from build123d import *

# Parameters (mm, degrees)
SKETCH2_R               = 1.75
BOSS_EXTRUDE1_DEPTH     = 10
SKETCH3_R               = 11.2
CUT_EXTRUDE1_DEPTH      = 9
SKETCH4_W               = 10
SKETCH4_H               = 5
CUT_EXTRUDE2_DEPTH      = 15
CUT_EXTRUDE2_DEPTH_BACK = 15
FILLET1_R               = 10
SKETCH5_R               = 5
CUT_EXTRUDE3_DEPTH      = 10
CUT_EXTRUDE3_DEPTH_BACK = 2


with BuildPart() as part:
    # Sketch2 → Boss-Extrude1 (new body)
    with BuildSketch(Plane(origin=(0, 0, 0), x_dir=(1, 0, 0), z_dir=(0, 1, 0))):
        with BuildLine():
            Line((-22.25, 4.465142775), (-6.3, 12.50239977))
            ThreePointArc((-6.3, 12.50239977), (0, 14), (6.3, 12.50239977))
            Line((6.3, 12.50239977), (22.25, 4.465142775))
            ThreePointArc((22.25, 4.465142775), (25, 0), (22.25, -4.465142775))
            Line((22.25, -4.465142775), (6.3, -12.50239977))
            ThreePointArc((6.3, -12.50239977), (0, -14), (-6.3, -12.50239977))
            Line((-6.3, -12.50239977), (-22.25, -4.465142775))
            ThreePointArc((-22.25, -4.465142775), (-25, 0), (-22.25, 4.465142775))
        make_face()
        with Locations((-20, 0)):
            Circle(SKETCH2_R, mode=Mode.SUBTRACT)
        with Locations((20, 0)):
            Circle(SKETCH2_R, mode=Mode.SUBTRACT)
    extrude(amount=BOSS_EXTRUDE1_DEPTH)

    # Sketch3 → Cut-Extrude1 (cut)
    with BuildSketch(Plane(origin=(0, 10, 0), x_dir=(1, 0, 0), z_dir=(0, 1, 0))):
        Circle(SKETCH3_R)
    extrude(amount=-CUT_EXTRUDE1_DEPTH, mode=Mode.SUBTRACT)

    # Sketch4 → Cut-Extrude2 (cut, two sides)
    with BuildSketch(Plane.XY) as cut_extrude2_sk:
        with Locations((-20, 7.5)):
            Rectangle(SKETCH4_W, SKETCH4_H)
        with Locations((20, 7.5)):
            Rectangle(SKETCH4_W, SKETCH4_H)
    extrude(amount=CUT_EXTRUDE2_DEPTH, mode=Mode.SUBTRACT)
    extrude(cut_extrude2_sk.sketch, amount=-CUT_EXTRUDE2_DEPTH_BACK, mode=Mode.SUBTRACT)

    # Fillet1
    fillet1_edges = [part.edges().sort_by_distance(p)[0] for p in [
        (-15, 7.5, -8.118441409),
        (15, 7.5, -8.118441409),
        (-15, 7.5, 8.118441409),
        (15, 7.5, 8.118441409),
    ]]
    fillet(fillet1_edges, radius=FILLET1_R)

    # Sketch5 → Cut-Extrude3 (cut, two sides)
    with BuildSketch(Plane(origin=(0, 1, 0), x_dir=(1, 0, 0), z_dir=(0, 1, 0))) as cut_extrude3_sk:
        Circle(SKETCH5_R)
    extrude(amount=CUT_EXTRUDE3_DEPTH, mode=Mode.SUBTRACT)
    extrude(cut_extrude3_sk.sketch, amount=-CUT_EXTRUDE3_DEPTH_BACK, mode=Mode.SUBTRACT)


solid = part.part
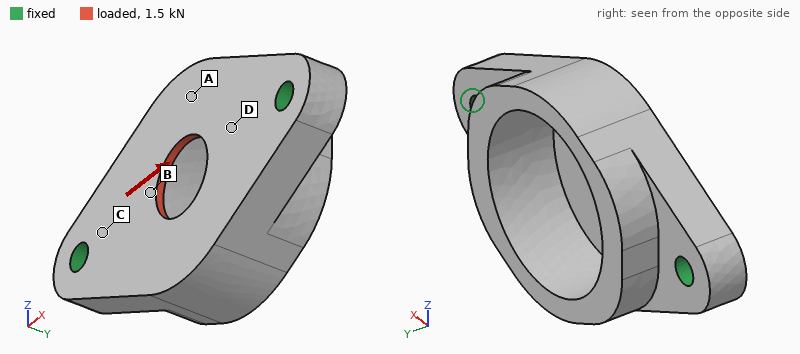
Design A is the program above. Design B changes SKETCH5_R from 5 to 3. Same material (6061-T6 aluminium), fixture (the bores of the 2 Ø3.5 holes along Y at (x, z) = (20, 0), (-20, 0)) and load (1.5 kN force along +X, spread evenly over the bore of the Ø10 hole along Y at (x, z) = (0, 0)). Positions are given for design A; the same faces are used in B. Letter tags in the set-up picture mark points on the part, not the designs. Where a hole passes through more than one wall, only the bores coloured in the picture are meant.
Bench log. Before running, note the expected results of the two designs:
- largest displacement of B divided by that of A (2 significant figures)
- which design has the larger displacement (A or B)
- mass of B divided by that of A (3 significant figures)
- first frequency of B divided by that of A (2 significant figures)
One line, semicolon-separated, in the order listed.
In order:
1.3; B; 1.01; 1.00
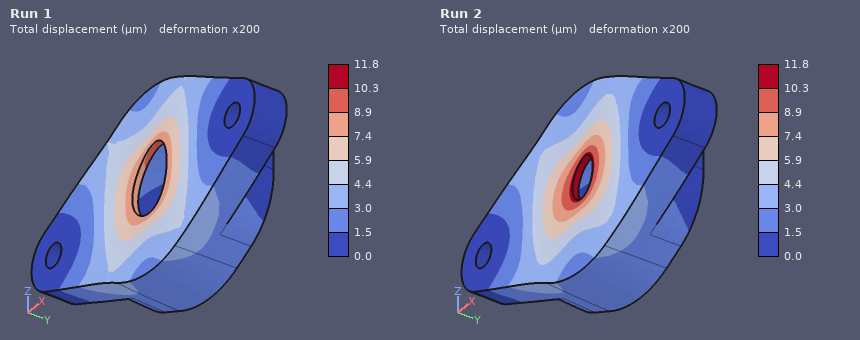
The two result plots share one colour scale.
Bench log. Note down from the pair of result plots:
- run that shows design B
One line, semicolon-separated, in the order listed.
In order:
Run 2
